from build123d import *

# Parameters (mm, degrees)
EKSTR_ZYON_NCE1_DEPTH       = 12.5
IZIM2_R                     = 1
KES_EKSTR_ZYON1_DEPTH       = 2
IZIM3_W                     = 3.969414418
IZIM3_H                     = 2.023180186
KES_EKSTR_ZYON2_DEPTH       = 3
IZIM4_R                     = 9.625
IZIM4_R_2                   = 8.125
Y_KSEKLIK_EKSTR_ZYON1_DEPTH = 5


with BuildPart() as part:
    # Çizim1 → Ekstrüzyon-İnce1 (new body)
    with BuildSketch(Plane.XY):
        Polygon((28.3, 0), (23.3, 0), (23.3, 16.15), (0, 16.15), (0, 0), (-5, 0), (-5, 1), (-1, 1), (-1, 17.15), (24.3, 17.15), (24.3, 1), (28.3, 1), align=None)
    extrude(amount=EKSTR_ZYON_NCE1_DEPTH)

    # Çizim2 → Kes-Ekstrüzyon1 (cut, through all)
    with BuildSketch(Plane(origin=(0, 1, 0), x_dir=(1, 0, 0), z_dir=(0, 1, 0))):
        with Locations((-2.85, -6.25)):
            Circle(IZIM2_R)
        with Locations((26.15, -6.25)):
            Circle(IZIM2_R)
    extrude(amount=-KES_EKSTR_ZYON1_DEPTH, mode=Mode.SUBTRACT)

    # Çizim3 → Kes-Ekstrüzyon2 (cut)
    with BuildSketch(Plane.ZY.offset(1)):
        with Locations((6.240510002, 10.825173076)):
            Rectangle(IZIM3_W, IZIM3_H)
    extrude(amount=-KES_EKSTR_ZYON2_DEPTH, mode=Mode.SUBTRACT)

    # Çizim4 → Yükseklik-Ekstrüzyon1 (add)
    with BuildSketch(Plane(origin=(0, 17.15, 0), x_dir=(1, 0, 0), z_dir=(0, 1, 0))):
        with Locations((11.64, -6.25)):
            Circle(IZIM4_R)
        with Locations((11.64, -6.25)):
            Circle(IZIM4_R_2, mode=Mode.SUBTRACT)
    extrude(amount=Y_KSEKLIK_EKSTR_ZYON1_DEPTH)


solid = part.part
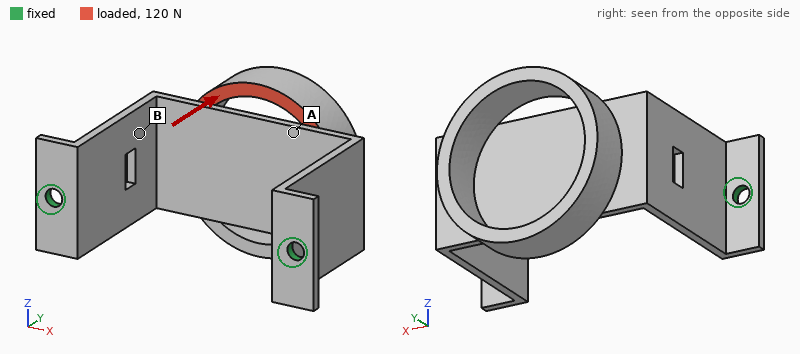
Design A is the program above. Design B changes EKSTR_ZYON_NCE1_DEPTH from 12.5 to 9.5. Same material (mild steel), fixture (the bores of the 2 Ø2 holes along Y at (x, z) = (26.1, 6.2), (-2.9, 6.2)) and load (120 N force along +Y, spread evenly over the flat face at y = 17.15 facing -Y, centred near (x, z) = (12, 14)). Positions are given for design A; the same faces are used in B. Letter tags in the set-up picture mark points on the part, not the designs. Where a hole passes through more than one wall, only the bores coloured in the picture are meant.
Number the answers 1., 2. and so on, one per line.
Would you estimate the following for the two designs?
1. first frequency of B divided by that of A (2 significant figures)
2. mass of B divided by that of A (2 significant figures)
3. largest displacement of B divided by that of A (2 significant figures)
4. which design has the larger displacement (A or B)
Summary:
1. 0.94
2. 0.84
3. 1.2
4. B
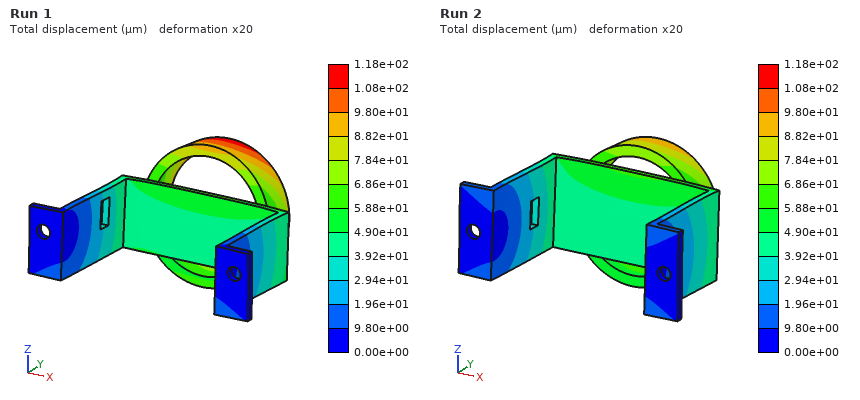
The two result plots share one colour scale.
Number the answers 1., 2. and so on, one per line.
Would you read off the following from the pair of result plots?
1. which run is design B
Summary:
1. Run 1
